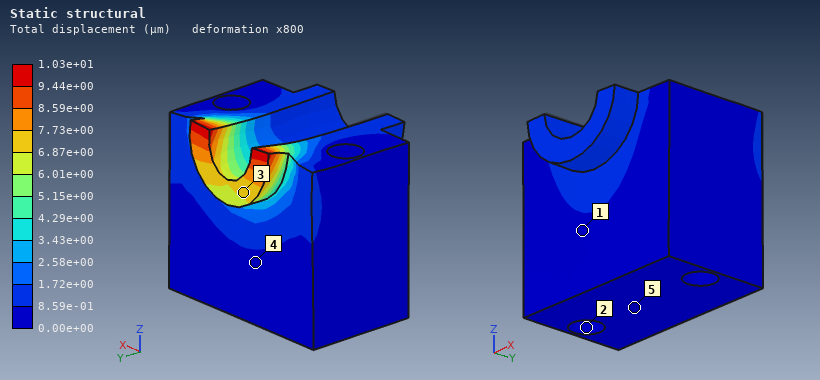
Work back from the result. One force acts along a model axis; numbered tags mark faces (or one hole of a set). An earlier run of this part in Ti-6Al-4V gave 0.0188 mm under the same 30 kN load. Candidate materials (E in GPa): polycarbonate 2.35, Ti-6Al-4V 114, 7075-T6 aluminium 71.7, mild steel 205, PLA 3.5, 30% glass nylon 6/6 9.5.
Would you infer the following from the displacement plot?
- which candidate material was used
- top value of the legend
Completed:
mild steel
1.03e+01 µm
